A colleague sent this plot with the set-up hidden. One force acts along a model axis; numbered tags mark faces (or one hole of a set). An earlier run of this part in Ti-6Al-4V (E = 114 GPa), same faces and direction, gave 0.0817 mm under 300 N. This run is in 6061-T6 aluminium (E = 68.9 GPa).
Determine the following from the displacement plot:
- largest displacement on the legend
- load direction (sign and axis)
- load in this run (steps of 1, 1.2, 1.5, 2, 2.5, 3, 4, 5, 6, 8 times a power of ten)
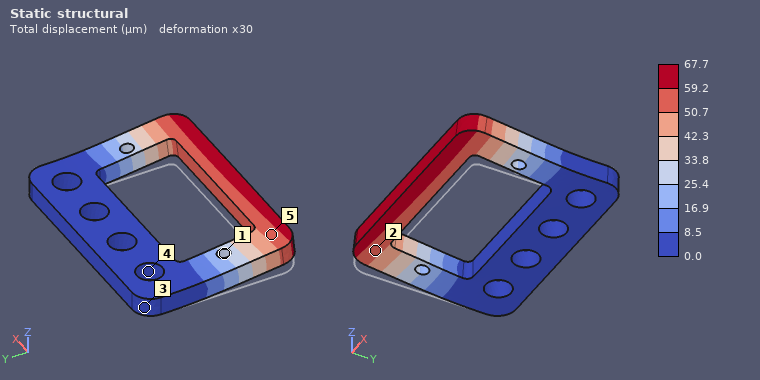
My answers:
67.7 µm
+Z
150 N
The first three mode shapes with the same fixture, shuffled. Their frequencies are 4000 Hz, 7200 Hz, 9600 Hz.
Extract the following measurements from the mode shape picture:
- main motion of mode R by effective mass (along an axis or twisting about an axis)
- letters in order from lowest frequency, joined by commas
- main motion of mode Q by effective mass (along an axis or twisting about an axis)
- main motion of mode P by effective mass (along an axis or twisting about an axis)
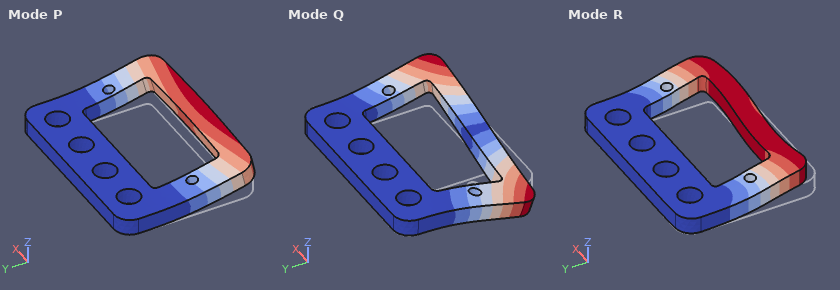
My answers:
along X
P, Q, R
twisting about Y
along Z
